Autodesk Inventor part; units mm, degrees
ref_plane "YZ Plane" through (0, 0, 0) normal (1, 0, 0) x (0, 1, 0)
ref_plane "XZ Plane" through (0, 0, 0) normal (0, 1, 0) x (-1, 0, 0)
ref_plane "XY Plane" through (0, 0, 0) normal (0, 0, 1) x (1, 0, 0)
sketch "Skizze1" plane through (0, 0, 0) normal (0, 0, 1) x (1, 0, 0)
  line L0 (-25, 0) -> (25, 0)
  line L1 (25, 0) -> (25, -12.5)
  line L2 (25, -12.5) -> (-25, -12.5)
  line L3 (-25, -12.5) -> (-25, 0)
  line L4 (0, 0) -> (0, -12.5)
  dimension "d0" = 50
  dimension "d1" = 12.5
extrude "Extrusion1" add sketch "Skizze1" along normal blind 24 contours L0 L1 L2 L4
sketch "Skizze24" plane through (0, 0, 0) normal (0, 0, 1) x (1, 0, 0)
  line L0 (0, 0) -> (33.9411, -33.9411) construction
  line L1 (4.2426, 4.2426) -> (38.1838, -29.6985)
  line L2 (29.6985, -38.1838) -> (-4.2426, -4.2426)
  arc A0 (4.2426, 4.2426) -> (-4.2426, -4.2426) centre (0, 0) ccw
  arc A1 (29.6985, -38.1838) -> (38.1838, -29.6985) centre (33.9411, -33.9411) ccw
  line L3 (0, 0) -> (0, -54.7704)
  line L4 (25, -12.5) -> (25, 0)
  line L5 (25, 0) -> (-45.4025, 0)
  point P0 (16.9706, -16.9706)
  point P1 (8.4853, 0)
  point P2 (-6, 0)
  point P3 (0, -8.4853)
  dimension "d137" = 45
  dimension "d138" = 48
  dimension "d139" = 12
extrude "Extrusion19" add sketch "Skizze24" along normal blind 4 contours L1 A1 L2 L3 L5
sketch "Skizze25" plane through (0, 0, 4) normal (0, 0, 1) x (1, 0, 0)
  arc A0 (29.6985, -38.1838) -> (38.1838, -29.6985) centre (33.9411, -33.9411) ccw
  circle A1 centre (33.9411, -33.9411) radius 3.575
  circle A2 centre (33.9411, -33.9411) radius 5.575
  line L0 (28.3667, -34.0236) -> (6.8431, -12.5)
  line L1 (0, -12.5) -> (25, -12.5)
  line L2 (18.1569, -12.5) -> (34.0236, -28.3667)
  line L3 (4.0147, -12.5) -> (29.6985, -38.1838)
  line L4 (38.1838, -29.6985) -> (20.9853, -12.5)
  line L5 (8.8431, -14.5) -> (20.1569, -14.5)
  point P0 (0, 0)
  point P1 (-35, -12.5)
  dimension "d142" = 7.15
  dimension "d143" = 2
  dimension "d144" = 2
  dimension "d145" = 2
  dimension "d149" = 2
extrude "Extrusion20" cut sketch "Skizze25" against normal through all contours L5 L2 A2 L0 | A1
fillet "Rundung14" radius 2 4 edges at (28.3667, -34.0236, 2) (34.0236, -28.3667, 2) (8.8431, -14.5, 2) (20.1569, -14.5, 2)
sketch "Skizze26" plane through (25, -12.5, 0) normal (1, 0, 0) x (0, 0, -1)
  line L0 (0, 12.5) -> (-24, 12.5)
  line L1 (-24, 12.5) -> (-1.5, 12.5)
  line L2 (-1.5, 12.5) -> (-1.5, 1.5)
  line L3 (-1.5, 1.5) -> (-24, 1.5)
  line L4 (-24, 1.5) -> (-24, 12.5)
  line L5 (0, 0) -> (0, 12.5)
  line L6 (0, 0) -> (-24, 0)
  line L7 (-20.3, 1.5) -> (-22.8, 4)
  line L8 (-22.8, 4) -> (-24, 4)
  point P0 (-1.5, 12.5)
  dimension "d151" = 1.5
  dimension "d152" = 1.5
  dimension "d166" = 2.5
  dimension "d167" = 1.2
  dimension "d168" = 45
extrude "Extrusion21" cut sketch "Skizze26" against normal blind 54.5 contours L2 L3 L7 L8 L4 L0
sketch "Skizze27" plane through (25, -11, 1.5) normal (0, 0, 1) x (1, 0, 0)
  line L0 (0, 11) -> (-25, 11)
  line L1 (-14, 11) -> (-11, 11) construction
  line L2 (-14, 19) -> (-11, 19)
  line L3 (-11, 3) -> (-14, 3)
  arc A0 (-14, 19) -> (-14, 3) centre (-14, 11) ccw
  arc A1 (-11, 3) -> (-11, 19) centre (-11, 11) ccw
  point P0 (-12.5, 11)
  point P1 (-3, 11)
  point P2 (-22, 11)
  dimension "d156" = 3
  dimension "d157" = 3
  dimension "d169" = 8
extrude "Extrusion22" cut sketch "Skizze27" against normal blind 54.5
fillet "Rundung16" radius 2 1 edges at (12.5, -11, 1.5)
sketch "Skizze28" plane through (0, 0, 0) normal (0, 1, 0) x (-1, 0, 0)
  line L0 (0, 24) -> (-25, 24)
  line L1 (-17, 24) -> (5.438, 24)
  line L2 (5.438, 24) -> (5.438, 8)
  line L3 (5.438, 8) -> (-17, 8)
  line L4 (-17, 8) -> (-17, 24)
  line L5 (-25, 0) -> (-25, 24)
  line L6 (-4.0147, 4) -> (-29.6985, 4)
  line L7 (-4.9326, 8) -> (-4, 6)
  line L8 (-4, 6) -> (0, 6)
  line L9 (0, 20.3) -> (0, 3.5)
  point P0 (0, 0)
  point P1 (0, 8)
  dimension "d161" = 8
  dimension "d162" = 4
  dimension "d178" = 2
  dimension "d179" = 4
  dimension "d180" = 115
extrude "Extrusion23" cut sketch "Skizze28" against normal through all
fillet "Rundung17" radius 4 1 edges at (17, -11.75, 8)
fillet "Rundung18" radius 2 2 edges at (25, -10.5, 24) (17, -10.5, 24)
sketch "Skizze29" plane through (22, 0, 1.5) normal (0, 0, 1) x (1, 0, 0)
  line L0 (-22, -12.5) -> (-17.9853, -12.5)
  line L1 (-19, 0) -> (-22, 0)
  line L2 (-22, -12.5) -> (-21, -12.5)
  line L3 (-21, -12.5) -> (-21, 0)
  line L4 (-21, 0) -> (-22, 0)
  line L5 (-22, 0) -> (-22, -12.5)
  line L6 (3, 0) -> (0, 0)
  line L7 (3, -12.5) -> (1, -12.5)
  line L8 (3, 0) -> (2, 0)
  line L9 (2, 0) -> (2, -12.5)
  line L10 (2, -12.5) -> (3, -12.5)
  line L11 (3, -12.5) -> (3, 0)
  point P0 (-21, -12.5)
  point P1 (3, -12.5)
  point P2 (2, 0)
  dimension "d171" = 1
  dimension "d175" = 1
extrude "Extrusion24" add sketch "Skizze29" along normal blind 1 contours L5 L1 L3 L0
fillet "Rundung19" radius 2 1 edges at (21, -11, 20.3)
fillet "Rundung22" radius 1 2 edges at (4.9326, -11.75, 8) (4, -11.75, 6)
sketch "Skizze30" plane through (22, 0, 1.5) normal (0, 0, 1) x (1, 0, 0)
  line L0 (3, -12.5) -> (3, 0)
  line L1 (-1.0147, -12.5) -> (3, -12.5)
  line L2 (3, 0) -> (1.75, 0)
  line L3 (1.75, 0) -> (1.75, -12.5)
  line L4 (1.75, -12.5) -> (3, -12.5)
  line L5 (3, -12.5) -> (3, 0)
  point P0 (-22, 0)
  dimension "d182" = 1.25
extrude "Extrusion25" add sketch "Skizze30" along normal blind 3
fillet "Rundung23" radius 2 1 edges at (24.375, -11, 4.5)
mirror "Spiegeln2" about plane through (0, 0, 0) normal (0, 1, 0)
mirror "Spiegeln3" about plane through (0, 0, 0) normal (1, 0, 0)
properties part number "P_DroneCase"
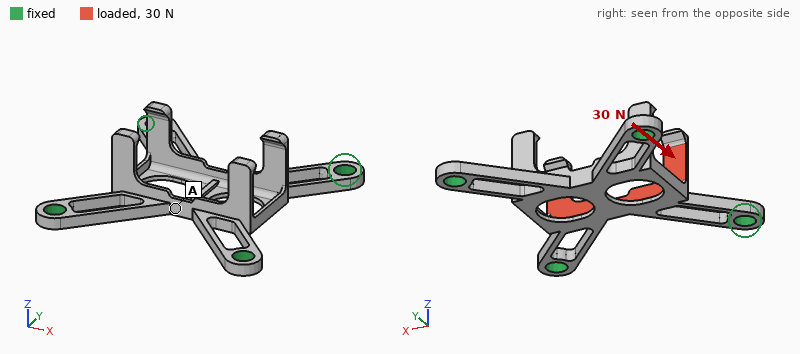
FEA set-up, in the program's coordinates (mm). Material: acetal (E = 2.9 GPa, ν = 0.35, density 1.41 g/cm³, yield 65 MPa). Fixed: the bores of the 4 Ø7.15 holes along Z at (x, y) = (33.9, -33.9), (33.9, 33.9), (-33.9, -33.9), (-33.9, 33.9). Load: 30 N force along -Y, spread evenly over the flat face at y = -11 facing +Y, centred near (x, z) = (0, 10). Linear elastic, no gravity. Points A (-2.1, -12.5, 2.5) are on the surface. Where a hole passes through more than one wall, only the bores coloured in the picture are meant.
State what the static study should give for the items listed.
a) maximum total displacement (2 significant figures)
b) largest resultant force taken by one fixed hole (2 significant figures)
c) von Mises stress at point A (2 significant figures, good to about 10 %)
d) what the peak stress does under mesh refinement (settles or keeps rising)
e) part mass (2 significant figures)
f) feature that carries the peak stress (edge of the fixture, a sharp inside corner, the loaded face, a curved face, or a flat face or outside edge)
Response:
1.1 mm
20 N
1.7 MPa
keeps rising
9.4 g
a sharp inside corner
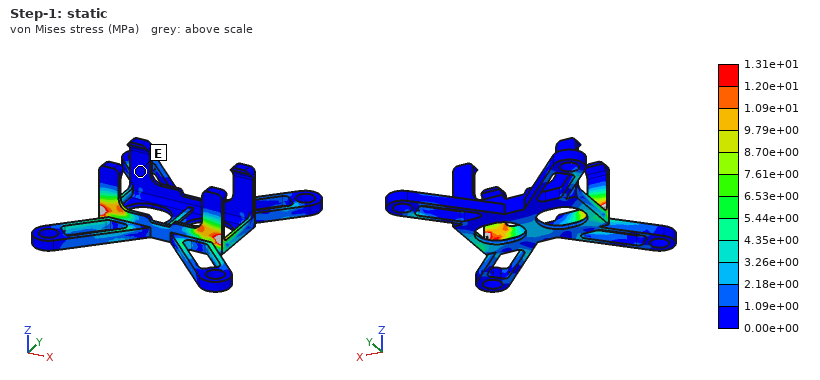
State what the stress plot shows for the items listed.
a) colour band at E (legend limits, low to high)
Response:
0.00e+00 to 1.09e+00 MPa
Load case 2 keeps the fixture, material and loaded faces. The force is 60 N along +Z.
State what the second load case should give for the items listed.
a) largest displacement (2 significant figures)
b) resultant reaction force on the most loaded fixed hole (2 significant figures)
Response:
1.2 mm
31 N
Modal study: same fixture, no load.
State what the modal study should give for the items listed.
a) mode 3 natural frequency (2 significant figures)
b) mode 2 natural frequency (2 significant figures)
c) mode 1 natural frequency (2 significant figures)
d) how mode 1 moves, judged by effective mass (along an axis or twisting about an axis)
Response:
700 Hz
640 Hz
550 Hz
along Z
